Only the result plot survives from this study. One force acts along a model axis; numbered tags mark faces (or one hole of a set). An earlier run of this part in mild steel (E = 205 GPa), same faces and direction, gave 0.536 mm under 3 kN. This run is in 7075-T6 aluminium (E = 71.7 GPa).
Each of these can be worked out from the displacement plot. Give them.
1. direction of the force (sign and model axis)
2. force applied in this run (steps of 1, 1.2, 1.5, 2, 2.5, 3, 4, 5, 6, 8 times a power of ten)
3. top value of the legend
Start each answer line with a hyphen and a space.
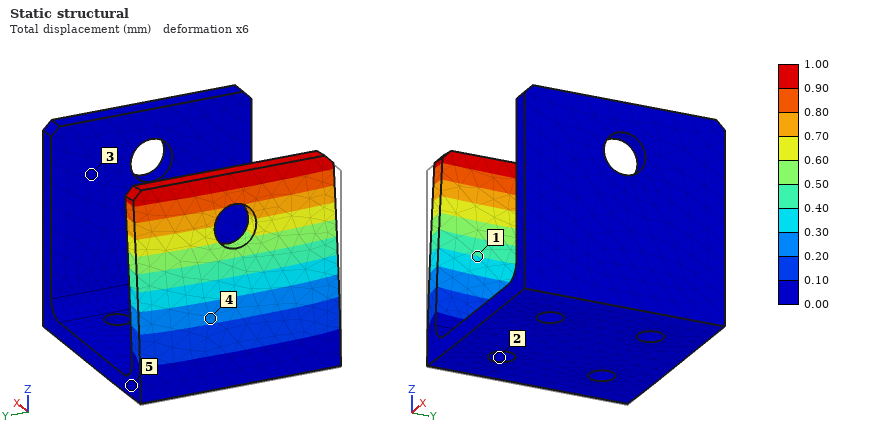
- +X
- 2 kN
- 1.00 mm
